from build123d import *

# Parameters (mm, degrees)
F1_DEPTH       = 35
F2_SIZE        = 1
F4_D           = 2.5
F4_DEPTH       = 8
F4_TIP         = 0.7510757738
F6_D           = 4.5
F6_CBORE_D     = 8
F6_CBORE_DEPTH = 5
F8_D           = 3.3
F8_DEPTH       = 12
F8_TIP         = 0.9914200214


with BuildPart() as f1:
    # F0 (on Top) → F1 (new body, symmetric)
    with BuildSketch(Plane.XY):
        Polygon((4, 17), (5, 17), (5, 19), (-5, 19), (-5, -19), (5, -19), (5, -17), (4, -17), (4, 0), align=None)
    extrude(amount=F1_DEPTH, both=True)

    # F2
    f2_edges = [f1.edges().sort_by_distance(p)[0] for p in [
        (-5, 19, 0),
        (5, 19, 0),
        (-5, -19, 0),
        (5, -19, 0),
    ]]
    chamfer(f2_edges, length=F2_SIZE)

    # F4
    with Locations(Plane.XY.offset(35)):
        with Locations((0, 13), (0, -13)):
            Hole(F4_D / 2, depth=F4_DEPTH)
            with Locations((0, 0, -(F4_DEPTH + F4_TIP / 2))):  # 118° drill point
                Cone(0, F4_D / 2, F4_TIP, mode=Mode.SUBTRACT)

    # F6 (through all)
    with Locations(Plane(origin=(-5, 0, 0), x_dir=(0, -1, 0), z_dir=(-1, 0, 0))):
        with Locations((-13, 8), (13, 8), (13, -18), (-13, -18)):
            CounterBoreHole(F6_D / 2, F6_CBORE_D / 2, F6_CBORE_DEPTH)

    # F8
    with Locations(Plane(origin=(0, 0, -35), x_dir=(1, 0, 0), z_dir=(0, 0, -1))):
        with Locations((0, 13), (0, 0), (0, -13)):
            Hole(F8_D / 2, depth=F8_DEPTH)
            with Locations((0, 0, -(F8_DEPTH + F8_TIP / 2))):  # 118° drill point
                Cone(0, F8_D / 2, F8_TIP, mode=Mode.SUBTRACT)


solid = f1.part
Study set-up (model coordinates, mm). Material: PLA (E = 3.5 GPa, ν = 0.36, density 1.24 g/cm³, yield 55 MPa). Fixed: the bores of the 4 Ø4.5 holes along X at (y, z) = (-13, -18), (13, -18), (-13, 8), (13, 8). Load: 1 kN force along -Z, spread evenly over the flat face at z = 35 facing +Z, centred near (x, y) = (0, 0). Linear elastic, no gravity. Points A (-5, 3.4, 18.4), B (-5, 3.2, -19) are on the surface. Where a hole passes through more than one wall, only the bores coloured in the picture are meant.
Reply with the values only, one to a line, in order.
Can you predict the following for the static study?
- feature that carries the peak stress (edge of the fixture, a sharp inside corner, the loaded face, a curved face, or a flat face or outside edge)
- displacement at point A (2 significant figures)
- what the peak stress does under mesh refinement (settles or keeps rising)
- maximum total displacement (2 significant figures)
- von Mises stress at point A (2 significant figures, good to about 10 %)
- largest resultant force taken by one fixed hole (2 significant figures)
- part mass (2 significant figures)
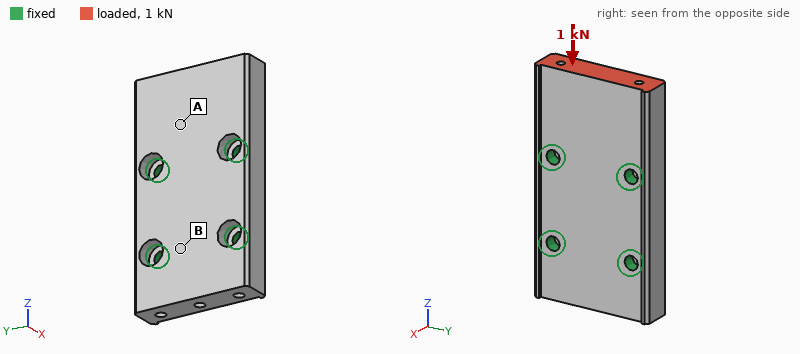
edge of the fixture
39 µm
keeps rising
79 µm
3.3 MPa
370 N
28 g
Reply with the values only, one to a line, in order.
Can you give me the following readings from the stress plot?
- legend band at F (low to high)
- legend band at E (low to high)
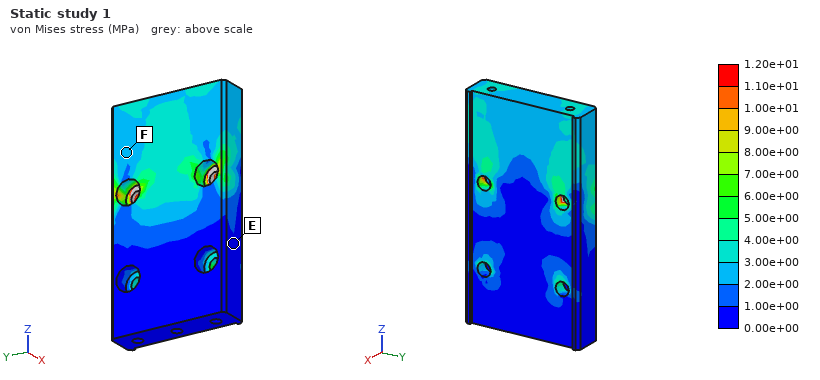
2.00e+00 to 3.00e+00 MPa
0.00e+00 to 1.00e+00 MPa
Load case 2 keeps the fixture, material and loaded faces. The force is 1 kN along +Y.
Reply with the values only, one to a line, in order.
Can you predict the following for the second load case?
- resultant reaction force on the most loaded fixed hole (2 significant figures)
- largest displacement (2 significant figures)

950 N
0.20 mm
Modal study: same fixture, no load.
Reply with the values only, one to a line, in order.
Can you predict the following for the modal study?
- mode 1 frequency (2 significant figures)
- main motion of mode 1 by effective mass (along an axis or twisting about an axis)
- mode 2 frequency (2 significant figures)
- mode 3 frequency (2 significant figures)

2300 Hz
along X
4600 Hz
4700 Hz
